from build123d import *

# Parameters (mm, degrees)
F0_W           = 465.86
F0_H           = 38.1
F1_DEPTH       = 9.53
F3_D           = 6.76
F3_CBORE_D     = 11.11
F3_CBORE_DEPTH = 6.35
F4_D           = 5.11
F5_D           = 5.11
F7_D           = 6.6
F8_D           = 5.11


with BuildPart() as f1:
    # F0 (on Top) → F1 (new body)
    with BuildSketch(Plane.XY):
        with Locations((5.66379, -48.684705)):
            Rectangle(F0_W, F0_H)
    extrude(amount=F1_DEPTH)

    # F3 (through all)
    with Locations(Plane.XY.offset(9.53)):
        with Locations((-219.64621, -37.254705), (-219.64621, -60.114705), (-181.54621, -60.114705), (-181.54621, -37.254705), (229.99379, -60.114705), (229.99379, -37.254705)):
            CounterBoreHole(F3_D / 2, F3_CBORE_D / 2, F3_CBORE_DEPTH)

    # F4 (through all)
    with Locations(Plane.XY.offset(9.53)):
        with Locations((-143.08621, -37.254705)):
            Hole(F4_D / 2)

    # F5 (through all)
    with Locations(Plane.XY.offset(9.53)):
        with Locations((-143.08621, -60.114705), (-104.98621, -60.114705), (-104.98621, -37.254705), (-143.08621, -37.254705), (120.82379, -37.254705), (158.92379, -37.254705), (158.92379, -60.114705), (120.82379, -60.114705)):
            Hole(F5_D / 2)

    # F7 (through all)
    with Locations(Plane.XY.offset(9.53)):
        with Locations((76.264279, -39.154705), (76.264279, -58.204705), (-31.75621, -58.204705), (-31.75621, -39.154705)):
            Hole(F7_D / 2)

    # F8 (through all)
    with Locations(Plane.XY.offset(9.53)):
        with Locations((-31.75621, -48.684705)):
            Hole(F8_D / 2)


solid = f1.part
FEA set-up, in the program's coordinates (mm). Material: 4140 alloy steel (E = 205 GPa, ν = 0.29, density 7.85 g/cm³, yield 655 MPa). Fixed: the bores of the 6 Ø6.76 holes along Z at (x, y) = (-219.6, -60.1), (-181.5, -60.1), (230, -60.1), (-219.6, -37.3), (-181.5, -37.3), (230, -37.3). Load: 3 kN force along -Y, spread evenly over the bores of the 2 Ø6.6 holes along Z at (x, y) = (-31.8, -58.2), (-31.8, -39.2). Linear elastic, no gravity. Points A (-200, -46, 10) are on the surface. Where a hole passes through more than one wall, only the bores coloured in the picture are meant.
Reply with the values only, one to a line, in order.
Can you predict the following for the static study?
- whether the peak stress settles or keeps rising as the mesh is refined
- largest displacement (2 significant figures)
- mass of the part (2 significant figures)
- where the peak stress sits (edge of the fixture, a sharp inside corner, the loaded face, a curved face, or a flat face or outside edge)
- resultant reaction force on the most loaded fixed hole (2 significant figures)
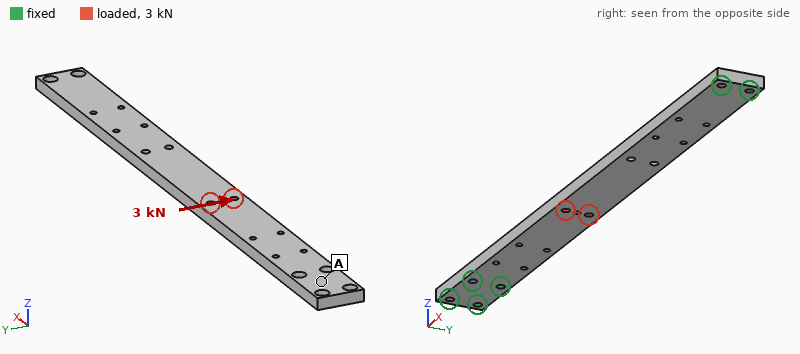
keeps rising
0.14 mm
1.3 kg
edge of the fixture
5.3 kN
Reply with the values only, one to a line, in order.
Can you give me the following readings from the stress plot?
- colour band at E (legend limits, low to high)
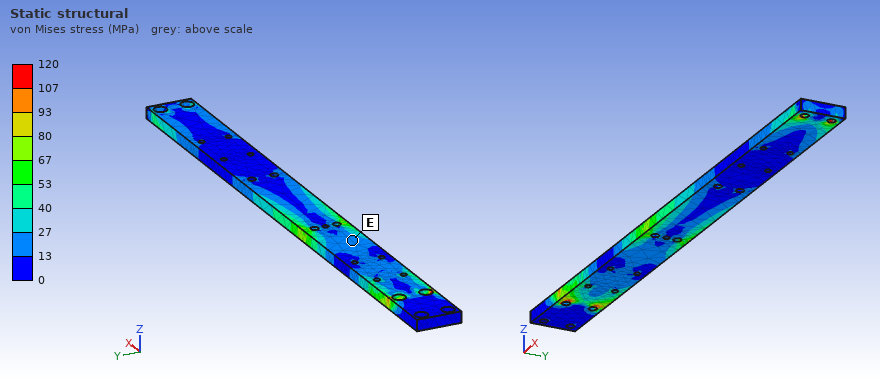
13 to 27 MPa
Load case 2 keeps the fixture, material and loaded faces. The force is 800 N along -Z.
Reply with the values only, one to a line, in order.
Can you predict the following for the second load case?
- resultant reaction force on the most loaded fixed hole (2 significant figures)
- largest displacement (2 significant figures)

1.7 kN
0.53 mm
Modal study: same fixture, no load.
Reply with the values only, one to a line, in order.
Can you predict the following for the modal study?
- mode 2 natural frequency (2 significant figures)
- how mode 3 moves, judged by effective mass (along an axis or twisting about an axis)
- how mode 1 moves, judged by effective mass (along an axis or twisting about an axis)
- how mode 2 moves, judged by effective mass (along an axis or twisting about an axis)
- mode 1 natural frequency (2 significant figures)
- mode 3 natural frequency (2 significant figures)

730 Hz
along Y
along Z
twisting about Y
270 Hz
1000 Hz
